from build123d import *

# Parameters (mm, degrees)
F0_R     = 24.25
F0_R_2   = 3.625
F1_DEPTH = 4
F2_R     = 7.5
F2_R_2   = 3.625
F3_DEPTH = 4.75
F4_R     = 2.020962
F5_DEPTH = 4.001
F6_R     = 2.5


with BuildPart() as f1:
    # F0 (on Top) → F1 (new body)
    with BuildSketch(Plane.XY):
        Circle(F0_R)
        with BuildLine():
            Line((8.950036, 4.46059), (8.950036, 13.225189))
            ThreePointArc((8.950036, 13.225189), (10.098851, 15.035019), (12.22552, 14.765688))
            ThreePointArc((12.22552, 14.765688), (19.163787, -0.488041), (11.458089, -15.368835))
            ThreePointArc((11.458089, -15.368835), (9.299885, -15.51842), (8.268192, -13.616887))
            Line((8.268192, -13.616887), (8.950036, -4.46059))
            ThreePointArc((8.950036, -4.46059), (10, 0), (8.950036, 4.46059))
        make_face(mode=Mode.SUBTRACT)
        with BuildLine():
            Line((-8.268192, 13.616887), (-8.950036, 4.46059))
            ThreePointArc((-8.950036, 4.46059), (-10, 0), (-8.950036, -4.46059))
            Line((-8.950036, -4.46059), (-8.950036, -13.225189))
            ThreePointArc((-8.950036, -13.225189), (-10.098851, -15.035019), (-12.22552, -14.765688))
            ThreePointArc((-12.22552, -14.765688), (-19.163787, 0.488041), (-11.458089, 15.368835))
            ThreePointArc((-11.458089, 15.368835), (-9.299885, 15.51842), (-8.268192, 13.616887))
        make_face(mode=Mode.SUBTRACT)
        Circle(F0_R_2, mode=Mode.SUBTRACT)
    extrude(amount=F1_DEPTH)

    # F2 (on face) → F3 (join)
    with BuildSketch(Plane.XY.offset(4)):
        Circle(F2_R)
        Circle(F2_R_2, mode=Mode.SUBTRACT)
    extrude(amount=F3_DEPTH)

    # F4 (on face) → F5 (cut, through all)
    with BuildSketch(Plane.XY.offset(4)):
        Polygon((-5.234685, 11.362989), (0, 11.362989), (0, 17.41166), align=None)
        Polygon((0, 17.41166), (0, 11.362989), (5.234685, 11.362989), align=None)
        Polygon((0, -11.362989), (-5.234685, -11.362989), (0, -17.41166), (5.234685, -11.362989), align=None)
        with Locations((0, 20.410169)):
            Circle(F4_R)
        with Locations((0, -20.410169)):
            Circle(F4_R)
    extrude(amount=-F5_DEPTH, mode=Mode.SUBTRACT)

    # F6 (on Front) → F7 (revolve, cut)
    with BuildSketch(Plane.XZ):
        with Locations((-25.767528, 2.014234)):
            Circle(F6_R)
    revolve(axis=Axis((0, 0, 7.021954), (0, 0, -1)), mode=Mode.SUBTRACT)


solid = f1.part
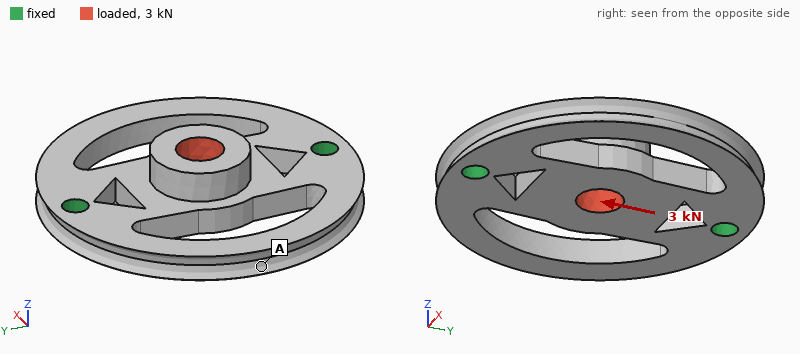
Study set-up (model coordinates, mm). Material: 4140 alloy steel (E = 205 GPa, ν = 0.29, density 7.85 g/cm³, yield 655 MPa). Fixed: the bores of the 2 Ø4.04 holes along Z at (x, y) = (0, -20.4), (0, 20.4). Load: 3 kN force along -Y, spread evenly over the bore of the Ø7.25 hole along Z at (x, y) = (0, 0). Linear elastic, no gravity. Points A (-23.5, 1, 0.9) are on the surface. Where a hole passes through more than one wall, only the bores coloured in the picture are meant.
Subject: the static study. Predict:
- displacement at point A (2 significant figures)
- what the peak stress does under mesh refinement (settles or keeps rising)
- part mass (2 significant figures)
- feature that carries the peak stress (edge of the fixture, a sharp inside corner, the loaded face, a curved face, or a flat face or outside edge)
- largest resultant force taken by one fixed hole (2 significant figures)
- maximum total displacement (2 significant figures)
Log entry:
3.4 µm
keeps rising
41 g
a sharp inside corner
1.5 kN
9.8 µm
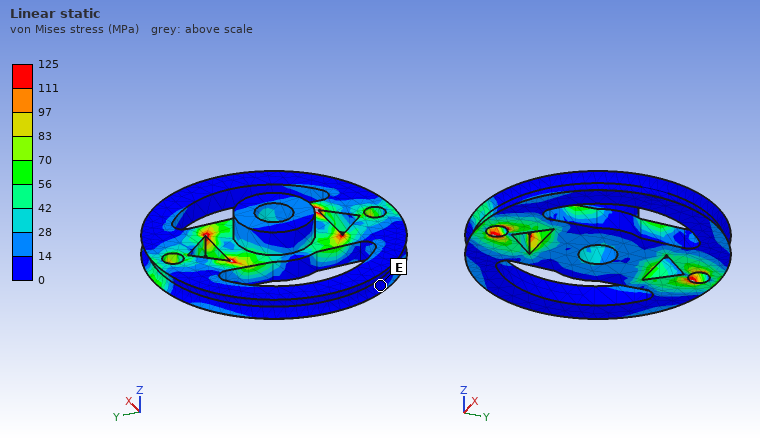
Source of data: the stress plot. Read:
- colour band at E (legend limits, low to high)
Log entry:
0 to 14 MPa
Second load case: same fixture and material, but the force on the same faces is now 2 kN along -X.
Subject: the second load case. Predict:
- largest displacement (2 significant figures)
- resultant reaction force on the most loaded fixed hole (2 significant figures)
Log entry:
22 µm
1.0 kN
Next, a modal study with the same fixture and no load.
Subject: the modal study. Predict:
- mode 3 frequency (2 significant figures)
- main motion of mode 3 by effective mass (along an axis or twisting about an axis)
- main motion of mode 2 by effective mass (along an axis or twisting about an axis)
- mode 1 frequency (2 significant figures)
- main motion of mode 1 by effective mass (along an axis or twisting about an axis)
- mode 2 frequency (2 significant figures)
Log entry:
11 kHz
along Z
along Z
5000 Hz
twisting about Y
5300 Hz
